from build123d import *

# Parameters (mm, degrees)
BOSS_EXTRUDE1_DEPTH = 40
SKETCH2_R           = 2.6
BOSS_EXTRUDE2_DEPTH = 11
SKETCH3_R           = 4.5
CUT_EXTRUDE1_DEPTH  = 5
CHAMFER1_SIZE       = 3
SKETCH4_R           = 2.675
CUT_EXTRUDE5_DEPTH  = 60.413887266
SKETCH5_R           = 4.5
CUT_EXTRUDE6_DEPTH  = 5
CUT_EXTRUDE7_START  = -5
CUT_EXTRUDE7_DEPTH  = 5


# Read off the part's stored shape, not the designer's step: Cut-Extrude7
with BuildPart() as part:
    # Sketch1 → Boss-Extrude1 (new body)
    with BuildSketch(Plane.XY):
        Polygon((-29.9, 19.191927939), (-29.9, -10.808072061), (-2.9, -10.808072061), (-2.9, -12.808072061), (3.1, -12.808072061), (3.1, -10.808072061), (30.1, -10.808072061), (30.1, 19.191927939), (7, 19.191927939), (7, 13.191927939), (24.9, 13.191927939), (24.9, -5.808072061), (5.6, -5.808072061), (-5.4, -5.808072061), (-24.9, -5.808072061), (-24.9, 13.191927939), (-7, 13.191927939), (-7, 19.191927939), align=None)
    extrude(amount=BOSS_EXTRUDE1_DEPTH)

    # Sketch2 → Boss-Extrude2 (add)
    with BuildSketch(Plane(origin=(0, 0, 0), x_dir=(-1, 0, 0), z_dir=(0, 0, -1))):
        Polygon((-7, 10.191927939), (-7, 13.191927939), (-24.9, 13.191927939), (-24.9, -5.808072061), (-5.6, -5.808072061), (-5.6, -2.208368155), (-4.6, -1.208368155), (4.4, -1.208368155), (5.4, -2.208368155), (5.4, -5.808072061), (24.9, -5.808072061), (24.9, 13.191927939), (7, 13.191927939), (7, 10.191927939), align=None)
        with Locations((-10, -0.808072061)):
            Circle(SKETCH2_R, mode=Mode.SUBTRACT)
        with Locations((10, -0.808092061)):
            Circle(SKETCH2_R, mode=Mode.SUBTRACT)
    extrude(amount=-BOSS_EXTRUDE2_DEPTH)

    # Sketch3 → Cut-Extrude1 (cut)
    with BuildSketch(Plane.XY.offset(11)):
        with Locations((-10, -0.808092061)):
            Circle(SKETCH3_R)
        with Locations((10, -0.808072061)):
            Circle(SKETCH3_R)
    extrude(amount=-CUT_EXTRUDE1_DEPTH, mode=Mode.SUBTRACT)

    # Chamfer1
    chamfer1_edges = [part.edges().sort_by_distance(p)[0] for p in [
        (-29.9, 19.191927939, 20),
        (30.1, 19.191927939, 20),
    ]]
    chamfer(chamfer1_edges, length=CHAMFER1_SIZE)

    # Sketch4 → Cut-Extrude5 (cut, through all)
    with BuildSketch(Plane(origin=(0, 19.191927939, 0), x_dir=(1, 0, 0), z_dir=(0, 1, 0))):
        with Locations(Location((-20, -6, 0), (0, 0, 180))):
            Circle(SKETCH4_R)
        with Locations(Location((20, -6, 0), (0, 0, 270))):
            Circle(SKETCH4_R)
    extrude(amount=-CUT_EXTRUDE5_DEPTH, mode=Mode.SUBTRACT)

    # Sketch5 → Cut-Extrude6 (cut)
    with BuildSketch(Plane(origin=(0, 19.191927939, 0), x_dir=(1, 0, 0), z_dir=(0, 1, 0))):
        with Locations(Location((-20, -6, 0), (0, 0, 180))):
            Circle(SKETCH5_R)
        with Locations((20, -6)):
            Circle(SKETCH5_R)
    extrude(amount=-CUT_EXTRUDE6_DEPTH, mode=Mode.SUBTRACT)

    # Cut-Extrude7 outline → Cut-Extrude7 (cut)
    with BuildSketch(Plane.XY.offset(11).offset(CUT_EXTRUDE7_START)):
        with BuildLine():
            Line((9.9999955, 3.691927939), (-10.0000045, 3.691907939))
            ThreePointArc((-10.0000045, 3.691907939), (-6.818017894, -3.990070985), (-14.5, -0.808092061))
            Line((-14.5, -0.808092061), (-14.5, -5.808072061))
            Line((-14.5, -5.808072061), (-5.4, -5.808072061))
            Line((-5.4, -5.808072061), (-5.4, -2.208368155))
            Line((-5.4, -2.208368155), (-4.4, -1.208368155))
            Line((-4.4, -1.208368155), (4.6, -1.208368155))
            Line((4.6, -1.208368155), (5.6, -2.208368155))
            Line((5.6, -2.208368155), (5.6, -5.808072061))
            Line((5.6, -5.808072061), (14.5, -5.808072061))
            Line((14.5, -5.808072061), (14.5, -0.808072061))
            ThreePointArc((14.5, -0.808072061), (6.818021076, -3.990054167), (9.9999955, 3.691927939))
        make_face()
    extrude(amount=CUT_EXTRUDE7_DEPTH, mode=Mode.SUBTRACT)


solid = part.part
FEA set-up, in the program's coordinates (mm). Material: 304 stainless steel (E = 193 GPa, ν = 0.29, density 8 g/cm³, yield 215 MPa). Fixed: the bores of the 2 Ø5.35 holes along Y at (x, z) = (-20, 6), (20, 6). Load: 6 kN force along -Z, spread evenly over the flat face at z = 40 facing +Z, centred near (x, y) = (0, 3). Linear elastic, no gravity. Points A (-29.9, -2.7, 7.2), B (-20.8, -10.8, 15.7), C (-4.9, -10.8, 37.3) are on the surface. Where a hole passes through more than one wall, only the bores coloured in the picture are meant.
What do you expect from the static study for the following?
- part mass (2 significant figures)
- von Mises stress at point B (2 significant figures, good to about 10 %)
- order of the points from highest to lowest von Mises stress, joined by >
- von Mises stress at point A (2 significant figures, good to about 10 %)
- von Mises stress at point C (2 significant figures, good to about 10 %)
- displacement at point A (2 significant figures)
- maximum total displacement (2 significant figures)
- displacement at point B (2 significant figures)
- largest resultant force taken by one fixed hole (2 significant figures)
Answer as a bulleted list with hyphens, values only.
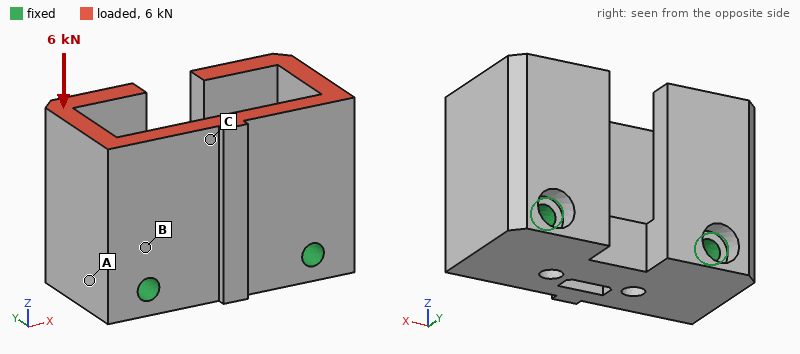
- 300 g
- 11 MPa
- B > C > A
- 3.3 MPa
- 7.6 MPa
- 0.54 µm
- 3.0 µm
- 0.56 µm
- 3.0 kN
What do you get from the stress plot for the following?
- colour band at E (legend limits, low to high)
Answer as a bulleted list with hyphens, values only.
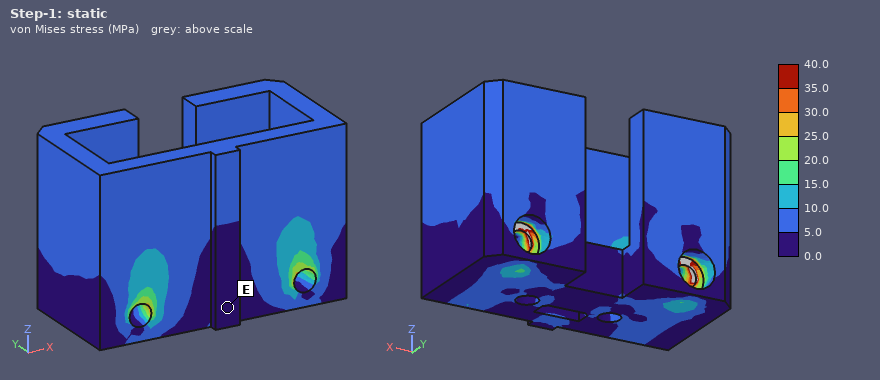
- 0.0 to 5.0 MPa
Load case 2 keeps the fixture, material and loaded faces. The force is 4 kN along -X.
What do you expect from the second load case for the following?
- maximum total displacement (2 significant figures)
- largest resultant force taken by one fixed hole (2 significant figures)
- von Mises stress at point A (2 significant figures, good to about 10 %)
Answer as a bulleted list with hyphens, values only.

- 21 µm
- 3.0 kN
- 13 MPa
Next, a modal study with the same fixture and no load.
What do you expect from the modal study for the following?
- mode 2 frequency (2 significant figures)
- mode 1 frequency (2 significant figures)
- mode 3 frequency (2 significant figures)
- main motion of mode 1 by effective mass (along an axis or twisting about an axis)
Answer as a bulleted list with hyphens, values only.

- 7900 Hz
- 6500 Hz
- 9000 Hz
- along Y
